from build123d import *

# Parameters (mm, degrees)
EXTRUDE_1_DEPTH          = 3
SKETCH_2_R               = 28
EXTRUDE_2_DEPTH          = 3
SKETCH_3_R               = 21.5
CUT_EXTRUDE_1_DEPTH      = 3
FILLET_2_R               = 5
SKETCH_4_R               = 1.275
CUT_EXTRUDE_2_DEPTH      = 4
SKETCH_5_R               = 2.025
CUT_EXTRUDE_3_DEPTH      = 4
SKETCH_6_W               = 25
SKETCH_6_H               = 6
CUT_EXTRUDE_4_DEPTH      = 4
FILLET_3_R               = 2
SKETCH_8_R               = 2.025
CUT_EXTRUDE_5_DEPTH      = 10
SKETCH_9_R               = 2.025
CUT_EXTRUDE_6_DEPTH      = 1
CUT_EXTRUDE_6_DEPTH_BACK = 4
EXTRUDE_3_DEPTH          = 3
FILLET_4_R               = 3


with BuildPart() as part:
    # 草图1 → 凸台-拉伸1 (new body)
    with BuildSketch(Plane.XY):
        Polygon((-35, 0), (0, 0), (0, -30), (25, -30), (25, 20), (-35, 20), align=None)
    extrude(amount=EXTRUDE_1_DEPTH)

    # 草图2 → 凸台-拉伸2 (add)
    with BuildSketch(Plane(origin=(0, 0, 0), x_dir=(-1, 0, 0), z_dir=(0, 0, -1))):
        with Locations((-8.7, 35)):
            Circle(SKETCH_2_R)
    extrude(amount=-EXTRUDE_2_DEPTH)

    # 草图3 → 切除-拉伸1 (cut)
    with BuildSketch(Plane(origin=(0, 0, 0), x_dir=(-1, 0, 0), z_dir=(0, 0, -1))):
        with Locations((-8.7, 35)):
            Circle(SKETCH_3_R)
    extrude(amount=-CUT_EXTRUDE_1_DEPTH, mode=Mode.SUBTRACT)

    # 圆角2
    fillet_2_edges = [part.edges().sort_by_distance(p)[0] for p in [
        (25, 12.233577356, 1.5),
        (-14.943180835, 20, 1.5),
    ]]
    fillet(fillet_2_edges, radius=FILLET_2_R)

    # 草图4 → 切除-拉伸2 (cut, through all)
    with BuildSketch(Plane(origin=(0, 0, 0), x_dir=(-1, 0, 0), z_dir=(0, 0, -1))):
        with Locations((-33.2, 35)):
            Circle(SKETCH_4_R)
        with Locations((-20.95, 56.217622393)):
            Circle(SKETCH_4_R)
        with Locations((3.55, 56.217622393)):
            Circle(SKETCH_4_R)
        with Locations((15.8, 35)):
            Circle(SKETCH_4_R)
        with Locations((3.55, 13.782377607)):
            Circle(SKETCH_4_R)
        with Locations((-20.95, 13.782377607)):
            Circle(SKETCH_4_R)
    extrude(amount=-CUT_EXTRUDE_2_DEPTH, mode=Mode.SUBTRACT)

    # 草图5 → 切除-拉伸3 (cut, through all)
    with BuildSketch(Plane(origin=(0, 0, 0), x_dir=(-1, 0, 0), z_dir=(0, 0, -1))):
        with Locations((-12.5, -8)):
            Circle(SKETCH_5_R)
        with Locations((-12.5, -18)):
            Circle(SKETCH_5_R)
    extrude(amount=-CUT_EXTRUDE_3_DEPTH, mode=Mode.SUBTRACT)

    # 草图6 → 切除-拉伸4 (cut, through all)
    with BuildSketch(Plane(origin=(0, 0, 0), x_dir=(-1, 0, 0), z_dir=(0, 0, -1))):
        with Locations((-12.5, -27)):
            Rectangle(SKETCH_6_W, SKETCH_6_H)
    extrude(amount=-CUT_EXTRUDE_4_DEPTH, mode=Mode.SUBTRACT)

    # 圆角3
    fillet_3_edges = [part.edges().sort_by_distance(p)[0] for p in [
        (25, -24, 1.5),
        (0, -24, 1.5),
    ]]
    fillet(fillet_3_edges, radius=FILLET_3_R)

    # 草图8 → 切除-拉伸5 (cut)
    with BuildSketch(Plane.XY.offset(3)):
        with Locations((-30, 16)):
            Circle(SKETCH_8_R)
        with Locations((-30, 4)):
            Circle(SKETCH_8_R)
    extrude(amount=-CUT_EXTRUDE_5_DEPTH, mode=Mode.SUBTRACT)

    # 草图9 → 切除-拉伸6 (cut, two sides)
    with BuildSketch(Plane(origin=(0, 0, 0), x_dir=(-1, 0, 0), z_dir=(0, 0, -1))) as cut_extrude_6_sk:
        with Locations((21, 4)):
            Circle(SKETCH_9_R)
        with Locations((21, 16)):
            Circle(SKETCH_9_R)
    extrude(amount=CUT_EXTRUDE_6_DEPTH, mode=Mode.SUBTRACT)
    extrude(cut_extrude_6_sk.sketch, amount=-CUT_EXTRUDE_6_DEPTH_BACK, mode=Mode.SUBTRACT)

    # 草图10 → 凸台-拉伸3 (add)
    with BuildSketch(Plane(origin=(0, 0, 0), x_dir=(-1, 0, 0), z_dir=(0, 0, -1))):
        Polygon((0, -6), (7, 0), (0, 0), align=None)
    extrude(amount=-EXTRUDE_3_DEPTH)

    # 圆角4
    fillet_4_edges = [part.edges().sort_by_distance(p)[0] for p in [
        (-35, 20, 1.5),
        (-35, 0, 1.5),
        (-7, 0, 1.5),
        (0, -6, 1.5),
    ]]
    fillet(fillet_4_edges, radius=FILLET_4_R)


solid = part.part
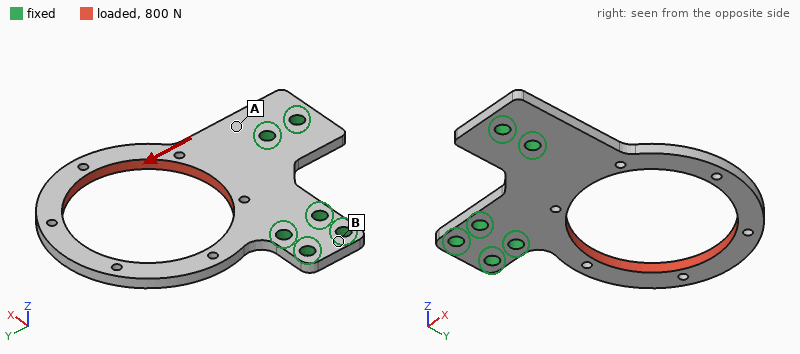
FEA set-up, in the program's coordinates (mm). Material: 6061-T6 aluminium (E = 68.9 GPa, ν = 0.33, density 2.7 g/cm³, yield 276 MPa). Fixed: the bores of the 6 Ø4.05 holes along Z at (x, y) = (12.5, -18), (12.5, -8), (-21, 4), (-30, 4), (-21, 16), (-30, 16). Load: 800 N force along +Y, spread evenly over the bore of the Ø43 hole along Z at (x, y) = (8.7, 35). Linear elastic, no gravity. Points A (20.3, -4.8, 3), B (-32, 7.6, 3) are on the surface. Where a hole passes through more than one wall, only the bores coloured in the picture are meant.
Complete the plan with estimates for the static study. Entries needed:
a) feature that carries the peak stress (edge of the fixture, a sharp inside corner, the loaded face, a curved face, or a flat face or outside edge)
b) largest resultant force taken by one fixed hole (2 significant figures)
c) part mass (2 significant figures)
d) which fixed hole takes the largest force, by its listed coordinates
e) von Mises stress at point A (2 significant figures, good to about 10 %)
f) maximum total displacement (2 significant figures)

a curved face
420 N
19 g
(12.5, -8)
12 MPa
99 µm
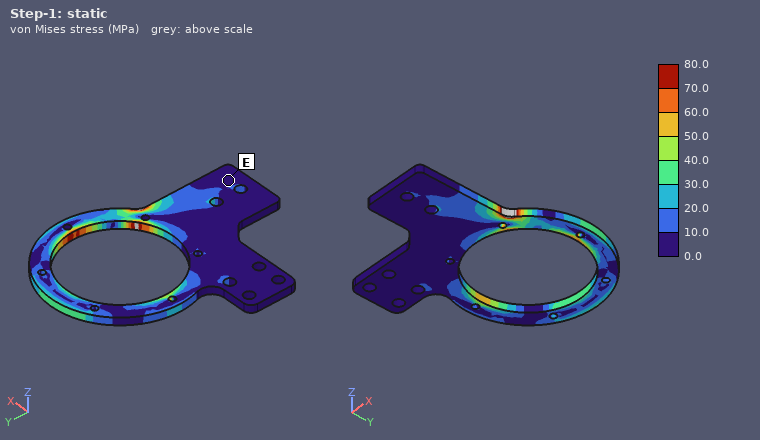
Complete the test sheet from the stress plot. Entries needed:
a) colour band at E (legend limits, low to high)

0.0 to 10.0 MPa
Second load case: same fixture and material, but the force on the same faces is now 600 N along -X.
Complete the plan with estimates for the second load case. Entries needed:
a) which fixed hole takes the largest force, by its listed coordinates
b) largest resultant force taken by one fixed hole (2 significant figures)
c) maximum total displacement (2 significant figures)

(-21, 16)
540 N
0.22 mm
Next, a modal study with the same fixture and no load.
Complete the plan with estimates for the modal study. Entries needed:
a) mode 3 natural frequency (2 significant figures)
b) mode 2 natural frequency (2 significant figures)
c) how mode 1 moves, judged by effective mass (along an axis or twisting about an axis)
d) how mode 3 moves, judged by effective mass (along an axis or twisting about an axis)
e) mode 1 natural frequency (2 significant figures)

3100 Hz
1700 Hz
along Z
along X
670 Hz
